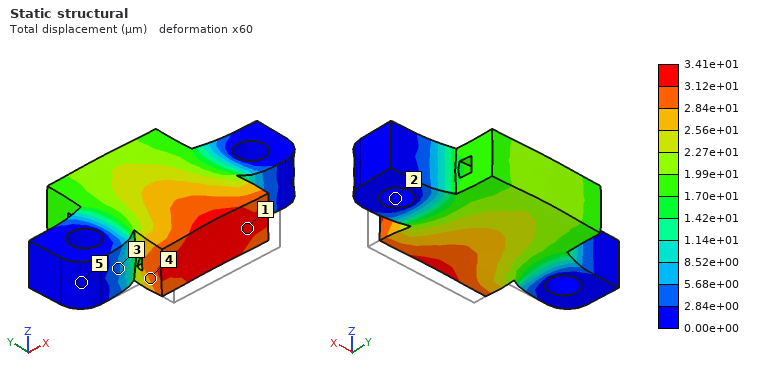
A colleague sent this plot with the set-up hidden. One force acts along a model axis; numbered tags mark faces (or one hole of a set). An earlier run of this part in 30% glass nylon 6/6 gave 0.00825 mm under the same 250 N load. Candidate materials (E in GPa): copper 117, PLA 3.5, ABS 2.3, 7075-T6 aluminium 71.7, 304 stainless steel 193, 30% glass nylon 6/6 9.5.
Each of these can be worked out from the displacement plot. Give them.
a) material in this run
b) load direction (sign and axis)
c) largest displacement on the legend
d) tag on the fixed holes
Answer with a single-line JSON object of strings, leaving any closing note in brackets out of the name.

{"material in this run": "ABS", "load direction": "+Y", "largest displacement on the legend": "3.41e+01 µm", "tag on the fixed holes": "2"}
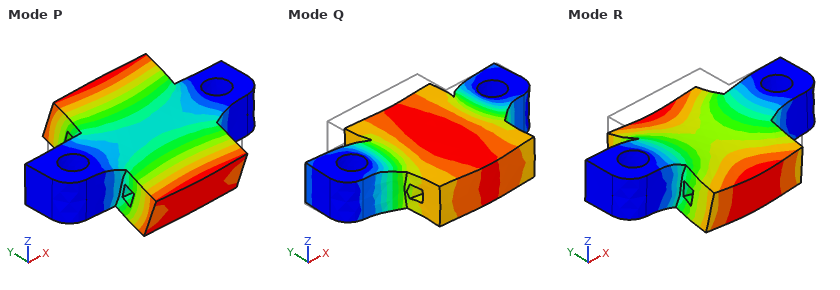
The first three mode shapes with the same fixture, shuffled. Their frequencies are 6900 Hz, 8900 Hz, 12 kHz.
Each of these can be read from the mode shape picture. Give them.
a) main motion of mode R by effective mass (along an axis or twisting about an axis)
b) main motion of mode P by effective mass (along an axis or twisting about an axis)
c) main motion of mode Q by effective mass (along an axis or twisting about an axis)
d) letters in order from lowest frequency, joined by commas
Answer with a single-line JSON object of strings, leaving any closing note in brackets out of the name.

{"main motion of mode R by effective mass": "along Z", "main motion of mode P by effective mass": "twisting about X", "main motion of mode Q by effective mass": "along Y", "letters in order from lowest frequency, joined by commas": "P, R, Q"}
